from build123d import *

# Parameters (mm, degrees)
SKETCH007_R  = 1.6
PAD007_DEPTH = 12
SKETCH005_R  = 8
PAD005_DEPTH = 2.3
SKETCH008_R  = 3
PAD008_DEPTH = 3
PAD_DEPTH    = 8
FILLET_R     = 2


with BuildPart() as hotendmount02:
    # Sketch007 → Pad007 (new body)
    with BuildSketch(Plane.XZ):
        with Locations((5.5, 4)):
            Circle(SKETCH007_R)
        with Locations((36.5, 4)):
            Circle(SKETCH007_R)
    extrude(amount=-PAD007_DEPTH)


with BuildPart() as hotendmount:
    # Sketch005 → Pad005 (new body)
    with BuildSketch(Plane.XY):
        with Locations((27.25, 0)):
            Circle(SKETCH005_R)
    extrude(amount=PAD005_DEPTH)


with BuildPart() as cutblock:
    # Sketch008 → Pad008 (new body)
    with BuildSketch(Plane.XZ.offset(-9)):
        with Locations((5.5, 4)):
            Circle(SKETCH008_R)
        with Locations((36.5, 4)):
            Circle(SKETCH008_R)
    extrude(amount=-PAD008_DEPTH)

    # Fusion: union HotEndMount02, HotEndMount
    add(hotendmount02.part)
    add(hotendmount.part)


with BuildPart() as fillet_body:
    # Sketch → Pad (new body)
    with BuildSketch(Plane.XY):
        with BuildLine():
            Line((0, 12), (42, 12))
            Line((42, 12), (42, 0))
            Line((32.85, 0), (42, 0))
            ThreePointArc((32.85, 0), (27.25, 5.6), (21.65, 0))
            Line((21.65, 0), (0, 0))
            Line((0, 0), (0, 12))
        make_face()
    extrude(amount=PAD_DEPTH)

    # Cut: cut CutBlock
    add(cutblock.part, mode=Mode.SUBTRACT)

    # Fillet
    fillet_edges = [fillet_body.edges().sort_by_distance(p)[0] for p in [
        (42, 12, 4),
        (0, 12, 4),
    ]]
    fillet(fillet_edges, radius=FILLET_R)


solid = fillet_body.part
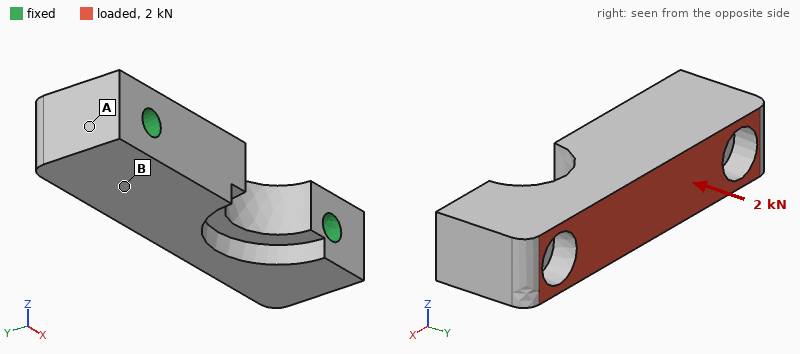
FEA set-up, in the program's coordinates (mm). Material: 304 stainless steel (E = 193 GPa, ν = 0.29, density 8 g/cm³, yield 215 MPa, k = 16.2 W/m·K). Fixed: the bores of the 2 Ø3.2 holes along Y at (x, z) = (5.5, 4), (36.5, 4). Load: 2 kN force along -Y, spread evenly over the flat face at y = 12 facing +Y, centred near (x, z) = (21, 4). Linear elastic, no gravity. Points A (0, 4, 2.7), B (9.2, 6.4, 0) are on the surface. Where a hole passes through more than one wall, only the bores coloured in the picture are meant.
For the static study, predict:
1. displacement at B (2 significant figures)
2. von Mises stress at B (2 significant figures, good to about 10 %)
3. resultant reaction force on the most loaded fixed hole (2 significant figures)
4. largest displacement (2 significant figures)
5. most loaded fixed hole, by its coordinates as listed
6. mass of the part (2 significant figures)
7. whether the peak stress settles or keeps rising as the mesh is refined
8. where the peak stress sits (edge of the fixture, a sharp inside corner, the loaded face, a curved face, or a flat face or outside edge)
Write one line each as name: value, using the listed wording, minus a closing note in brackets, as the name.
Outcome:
displacement at B: 0.82 µm
von Mises stress at B: 22 MPa
resultant reaction force on the most loaded fixed hole: 1.2 kN
largest displacement: 3.6 µm
most loaded fixed hole, by its coordinates as listed: (5.5, 4)
mass of the part: 26 g
whether the peak stress settles or keeps rising as the mesh is refined: keeps rising
where the peak stress sits: edge of the fixture
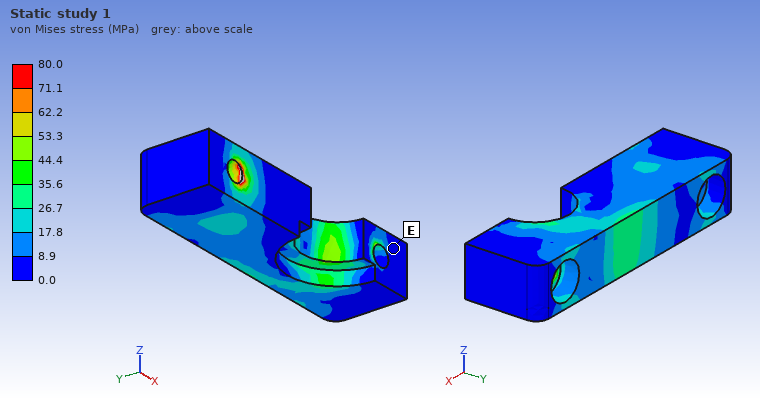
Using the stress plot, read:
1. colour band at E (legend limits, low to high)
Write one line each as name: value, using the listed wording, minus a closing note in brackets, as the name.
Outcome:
colour band at E: 0.0 to 8.9 MPa
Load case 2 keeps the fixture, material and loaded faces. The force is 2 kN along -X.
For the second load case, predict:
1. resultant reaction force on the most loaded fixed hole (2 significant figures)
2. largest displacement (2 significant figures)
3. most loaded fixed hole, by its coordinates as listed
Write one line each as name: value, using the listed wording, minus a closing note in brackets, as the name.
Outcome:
resultant reaction force on the most loaded fixed hole: 1.2 kN
largest displacement: 1.3 µm
most loaded fixed hole, by its coordinates as listed: (5.5, 4)
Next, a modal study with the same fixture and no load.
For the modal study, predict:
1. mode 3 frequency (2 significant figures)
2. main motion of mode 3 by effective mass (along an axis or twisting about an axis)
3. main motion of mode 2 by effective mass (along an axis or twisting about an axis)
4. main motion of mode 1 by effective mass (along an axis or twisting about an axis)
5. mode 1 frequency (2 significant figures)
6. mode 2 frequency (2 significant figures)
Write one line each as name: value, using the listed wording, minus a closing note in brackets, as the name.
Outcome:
mode 3 frequency: 39 kHz
main motion of mode 3 by effective mass: twisting about X
main motion of mode 2 by effective mass: along Y
main motion of mode 1 by effective mass: along Z
mode 1 frequency: 25 kHz
mode 2 frequency: 33 kHz
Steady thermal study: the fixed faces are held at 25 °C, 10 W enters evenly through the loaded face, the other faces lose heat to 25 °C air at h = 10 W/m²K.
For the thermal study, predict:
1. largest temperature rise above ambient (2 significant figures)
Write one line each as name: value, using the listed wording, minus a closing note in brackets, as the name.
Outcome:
largest temperature rise above ambient: 43 K
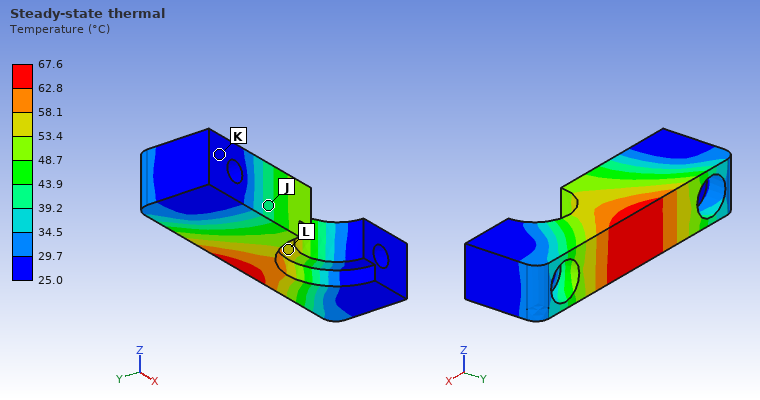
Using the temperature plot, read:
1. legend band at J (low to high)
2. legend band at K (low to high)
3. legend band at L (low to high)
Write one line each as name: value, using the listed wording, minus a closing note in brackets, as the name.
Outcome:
legend band at J: 39.2 to 43.9 °C
legend band at K: 25.0 to 29.7 °C
legend band at L: 53.4 to 58.1 °C
